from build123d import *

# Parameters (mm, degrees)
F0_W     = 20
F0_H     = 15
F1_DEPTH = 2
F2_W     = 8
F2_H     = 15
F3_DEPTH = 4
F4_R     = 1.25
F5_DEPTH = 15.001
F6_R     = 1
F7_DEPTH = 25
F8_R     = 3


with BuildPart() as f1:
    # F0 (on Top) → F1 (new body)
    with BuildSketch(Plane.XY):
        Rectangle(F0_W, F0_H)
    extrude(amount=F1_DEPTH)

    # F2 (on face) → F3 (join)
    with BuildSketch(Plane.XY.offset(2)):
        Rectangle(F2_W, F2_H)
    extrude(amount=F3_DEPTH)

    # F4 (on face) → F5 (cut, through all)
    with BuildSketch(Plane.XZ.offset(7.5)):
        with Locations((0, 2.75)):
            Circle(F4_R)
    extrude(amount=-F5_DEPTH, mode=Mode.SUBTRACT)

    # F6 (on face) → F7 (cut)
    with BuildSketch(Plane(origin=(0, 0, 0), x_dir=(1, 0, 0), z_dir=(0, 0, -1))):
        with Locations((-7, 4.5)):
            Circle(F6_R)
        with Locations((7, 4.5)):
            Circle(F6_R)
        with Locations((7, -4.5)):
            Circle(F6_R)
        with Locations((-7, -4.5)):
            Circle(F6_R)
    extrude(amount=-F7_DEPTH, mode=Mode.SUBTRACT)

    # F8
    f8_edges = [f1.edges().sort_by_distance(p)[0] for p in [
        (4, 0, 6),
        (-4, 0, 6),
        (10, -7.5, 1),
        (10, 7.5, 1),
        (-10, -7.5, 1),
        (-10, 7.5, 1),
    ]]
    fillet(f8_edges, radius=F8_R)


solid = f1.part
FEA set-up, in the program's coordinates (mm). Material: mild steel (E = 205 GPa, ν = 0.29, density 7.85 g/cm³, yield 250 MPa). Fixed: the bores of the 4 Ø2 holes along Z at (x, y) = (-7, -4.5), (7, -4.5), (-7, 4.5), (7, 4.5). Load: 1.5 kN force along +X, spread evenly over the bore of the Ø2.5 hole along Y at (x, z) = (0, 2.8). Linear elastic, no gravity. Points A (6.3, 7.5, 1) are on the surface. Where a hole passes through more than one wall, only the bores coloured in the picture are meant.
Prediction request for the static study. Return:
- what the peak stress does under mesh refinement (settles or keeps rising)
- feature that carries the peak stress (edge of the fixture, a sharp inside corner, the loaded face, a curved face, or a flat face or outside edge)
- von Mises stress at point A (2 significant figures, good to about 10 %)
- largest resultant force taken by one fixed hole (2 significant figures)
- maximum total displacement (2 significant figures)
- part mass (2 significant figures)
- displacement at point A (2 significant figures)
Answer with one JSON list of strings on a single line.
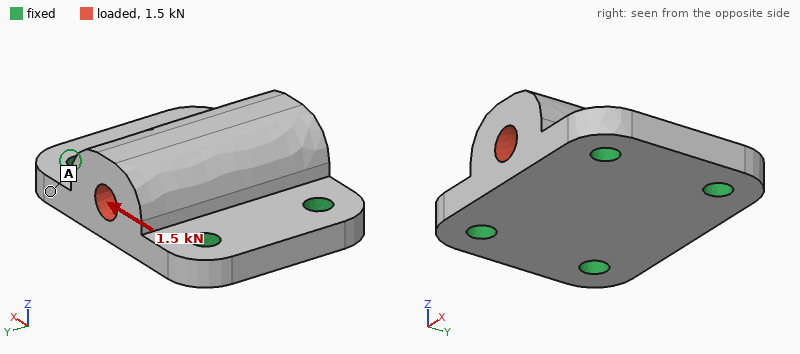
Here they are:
["keeps rising", "edge of the fixture", "15 MPa", "400 N", "1.6 µm", "7.1 g", "0.39 µm"]
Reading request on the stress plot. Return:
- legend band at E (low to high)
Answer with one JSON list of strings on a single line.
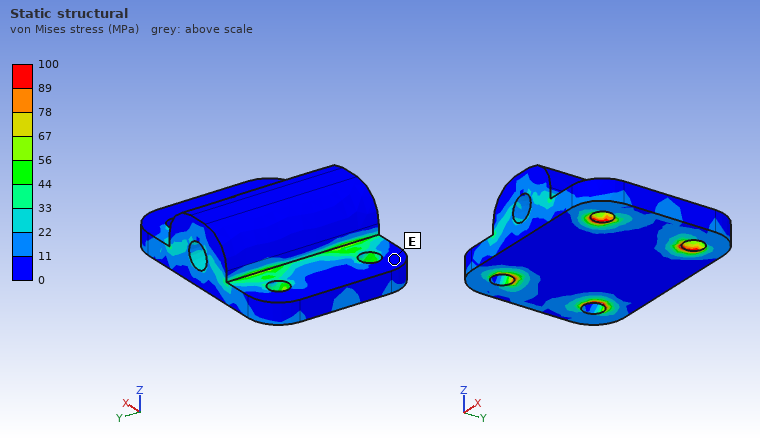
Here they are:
["0 to 11 MPa"]
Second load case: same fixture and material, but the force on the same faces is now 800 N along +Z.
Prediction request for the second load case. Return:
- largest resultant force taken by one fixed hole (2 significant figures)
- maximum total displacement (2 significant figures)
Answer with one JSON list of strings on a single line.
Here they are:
["210 N", "2.3 µm"]
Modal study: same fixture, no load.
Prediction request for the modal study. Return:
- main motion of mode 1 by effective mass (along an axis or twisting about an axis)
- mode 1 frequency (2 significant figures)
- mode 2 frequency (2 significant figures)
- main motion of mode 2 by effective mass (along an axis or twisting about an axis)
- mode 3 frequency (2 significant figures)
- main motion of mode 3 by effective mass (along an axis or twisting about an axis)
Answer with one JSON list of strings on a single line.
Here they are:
["along Y", "45 kHz", "48 kHz", "along Z", "72 kHz", "along X"]
